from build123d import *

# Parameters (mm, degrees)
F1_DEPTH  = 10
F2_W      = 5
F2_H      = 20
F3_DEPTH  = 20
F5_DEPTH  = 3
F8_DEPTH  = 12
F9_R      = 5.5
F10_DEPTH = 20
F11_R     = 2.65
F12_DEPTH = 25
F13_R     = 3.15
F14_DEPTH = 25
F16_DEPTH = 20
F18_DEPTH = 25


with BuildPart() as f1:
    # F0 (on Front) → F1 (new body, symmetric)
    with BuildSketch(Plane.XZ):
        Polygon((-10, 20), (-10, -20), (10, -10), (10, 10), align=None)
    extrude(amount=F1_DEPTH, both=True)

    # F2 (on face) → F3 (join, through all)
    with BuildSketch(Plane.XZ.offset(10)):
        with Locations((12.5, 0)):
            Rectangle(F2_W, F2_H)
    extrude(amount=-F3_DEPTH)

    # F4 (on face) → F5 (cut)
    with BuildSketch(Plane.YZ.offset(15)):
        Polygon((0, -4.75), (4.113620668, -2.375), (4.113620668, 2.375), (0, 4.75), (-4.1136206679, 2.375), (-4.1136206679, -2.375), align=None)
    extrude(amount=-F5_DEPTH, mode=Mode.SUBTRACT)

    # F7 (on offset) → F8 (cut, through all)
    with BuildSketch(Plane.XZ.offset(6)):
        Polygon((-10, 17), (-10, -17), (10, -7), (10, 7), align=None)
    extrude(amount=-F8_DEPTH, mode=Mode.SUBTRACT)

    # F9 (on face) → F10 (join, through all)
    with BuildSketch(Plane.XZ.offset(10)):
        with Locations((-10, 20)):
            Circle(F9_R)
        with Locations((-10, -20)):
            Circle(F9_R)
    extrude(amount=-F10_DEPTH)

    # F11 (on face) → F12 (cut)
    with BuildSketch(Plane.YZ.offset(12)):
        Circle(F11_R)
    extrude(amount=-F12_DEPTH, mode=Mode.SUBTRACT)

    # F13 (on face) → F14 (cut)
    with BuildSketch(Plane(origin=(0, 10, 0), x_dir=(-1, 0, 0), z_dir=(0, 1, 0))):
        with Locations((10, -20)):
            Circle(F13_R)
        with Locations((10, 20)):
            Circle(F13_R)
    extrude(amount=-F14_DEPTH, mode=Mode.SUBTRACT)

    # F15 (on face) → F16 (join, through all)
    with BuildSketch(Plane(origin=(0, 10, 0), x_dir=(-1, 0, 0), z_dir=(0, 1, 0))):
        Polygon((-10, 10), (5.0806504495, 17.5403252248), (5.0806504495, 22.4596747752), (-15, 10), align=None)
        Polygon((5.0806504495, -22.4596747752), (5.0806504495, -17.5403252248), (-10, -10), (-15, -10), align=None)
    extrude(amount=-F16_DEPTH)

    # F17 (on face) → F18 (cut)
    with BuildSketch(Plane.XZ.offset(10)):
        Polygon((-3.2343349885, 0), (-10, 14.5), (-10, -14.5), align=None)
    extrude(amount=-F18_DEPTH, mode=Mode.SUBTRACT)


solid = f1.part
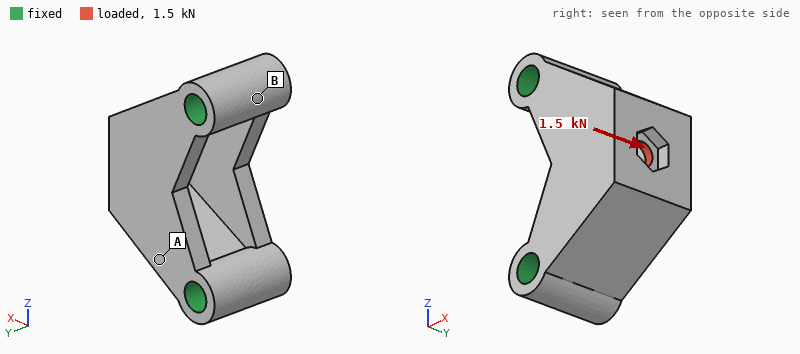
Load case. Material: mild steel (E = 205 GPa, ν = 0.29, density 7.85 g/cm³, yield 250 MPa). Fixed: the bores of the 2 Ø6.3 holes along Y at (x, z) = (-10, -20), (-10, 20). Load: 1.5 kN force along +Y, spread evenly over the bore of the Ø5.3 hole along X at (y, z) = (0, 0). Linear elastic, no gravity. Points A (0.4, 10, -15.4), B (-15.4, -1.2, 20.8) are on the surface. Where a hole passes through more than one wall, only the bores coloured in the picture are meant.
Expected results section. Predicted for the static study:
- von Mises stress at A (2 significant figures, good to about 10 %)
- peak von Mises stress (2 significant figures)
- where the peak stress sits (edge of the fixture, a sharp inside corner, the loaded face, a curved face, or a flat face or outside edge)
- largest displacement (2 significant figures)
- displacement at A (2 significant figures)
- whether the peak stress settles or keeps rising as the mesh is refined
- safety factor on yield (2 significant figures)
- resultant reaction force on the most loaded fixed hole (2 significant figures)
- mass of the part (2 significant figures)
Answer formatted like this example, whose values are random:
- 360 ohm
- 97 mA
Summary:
- 16 MPa
- 79 MPa
- the loaded face
- 5.2 µm
- 1.6 µm
- settles
- 3.2
- 750 N
- 93 g
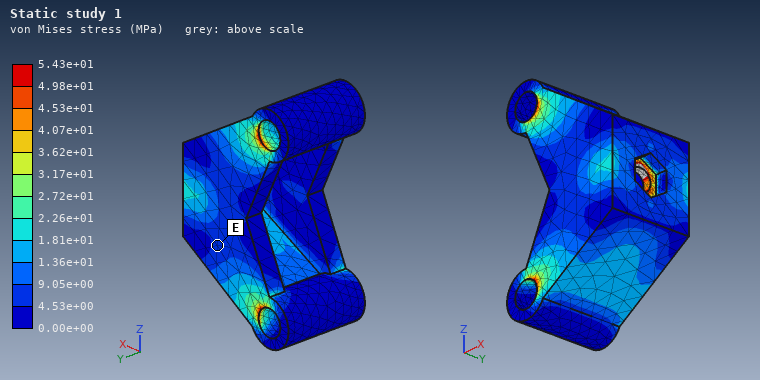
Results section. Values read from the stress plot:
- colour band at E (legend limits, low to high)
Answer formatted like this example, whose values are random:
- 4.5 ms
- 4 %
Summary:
- 4.53e+00 to 9.05e+00 MPa
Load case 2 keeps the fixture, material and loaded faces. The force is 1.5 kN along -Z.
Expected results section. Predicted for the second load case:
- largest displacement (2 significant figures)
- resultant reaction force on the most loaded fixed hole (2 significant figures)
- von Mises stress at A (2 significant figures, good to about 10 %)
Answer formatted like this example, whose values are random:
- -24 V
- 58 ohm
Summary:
- 2.5 µm
- 1.0 kN
- 5.5 MPa
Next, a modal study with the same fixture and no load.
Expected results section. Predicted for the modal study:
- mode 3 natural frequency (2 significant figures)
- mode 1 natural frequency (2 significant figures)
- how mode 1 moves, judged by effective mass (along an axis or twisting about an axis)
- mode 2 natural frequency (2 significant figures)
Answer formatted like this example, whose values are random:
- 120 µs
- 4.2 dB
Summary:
- 28 kHz
- 17 kHz
- along Y
- 27 kHz
